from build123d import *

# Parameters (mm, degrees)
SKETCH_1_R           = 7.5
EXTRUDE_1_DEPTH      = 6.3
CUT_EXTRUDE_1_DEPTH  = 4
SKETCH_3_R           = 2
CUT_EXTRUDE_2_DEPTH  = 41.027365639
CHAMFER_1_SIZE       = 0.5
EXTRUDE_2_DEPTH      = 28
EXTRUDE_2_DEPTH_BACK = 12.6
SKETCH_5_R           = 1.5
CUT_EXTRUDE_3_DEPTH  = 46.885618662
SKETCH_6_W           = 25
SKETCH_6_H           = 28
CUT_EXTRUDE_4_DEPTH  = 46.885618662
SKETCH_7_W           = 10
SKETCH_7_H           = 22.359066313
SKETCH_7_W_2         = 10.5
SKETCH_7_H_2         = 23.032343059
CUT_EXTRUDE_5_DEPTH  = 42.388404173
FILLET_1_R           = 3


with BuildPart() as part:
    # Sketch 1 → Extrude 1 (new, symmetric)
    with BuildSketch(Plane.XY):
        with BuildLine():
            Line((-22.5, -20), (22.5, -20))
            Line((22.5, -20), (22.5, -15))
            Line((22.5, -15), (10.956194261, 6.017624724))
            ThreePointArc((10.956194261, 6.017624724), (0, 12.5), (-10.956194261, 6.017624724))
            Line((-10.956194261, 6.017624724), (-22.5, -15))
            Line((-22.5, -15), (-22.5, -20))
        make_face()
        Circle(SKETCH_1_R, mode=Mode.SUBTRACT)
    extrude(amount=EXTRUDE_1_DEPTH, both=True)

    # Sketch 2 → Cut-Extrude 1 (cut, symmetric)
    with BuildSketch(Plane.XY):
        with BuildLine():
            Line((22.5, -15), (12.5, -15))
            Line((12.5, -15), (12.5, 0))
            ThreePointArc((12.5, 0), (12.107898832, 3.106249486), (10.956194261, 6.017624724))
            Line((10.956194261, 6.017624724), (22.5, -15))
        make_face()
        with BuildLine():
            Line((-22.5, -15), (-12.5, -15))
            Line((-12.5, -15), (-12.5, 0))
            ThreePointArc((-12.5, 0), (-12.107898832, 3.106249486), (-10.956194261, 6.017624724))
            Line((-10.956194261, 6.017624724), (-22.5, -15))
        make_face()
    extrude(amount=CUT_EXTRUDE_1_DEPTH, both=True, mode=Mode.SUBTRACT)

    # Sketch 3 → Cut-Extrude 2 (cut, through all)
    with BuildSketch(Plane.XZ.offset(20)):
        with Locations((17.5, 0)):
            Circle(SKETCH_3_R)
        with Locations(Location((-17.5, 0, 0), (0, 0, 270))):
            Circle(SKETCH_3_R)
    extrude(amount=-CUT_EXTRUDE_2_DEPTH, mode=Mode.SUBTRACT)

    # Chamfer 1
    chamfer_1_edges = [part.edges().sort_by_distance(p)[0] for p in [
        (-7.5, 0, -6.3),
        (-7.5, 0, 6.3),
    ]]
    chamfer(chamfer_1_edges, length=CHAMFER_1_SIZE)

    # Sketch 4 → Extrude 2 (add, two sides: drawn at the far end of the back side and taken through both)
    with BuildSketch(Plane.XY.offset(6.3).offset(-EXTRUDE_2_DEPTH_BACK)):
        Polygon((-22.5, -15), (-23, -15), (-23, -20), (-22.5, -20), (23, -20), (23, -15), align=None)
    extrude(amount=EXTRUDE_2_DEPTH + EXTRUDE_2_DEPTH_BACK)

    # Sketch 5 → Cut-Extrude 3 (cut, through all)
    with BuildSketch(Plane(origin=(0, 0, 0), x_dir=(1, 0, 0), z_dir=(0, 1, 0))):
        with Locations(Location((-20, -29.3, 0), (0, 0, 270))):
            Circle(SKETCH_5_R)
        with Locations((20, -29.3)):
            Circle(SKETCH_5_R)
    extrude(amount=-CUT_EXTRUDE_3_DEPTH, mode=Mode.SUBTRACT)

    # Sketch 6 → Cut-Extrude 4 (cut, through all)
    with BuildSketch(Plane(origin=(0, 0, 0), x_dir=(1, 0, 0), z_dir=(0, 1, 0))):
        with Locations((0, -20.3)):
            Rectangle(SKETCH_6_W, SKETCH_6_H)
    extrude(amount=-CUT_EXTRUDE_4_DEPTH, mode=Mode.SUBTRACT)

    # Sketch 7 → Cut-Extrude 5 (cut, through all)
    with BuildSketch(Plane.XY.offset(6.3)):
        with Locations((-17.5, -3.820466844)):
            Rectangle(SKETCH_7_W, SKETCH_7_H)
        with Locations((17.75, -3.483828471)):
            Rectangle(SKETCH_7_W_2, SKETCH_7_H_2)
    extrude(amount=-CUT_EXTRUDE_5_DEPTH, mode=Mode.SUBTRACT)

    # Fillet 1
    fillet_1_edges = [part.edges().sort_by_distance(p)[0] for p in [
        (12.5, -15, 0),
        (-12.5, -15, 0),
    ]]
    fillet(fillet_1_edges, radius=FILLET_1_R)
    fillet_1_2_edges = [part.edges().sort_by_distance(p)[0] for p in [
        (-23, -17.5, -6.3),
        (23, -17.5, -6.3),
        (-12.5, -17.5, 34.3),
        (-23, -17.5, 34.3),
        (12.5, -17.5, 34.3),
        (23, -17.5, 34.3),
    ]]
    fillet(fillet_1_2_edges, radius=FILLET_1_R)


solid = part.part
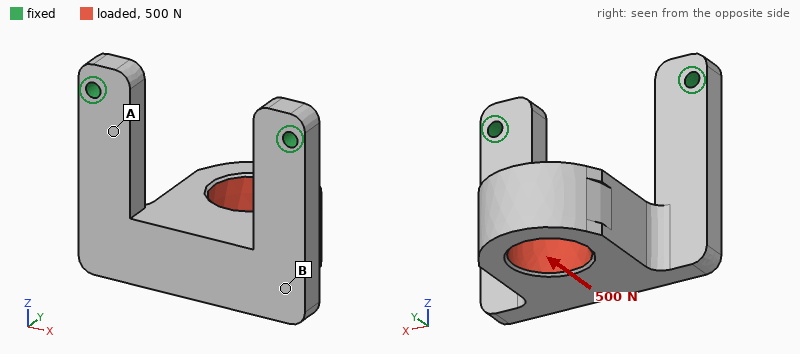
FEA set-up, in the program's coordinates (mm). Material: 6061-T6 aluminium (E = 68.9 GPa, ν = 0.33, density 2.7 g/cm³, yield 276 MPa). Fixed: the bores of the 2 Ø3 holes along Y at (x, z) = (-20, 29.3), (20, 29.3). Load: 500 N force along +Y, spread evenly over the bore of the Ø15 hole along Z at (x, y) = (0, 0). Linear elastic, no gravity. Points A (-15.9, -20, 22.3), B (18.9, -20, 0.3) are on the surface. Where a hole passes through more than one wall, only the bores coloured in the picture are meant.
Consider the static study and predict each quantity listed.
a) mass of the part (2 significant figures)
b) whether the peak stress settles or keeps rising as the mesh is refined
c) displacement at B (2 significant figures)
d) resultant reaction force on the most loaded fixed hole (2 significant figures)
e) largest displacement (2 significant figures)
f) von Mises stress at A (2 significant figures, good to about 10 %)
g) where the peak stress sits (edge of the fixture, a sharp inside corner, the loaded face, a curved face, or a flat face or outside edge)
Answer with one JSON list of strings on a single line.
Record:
["31 g", "keeps rising", "0.29 mm", "250 N", "0.58 mm", "120 MPa", "edge of the fixture"]
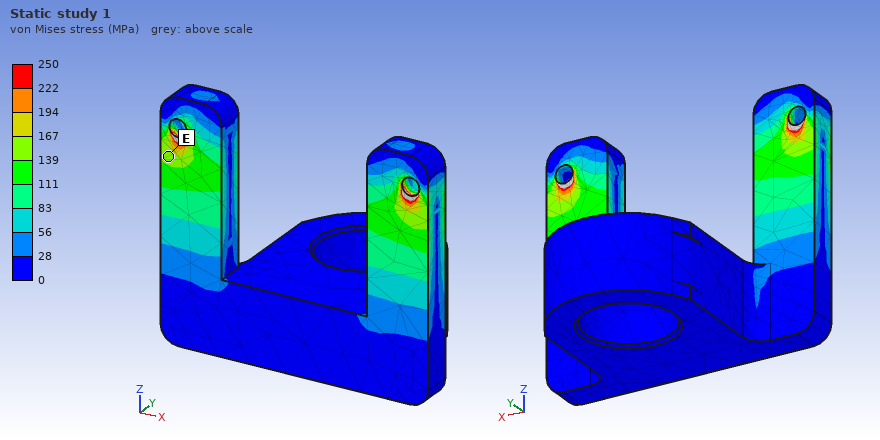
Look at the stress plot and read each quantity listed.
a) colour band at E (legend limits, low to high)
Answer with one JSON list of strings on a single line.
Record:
["139 to 167 MPa"]
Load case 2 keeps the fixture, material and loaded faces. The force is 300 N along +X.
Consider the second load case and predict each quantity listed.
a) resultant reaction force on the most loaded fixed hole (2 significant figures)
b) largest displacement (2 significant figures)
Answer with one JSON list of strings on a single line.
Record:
["250 N", "79 µm"]
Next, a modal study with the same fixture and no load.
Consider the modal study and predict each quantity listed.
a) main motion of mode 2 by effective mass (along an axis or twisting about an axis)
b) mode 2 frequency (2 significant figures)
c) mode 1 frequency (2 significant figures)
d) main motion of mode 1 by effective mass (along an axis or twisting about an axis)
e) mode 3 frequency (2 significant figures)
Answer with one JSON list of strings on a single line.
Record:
["along X", "2900 Hz", "1100 Hz", "along Y", "4100 Hz"]
